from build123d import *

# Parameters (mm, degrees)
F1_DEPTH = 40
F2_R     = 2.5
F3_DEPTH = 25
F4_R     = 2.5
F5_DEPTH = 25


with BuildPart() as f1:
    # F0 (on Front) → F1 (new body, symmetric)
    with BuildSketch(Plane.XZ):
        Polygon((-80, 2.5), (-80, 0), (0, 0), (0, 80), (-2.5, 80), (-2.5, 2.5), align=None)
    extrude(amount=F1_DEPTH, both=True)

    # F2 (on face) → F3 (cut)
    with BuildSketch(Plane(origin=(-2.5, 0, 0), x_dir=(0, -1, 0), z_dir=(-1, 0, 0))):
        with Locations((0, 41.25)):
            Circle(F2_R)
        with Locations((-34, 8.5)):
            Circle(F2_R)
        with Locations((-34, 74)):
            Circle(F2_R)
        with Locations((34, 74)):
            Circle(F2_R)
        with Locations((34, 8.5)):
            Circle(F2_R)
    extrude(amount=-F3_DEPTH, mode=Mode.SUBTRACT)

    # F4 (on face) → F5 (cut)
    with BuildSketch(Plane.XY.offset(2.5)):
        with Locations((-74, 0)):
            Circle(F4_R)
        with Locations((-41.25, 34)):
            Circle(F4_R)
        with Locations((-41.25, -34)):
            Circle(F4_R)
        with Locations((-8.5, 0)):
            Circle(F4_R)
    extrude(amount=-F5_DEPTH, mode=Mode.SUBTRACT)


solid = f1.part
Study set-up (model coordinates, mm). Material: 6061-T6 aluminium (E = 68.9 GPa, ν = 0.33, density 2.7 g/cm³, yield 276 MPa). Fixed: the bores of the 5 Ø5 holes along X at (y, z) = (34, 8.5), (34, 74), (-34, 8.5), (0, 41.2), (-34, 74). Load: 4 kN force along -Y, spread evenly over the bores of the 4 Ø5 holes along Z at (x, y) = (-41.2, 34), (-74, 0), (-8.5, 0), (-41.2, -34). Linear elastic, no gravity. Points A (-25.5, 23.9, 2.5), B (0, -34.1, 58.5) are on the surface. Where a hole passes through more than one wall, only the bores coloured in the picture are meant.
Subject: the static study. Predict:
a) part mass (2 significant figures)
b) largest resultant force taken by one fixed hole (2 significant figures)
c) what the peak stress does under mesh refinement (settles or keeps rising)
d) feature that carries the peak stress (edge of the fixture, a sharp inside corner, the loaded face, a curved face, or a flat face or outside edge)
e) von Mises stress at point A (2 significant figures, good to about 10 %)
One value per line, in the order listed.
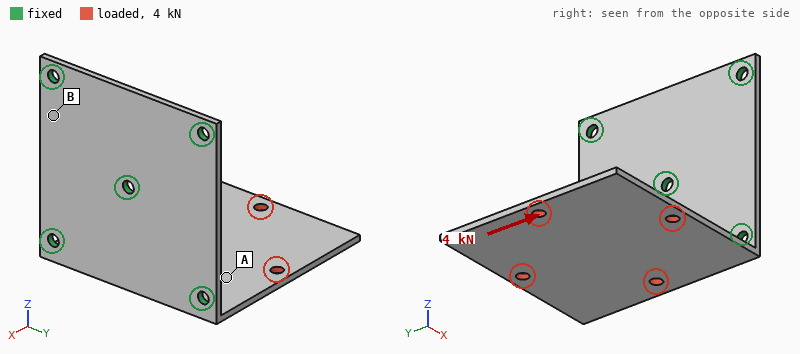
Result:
84 g
3.0 kN
keeps rising
edge of the fixture
58 MPa
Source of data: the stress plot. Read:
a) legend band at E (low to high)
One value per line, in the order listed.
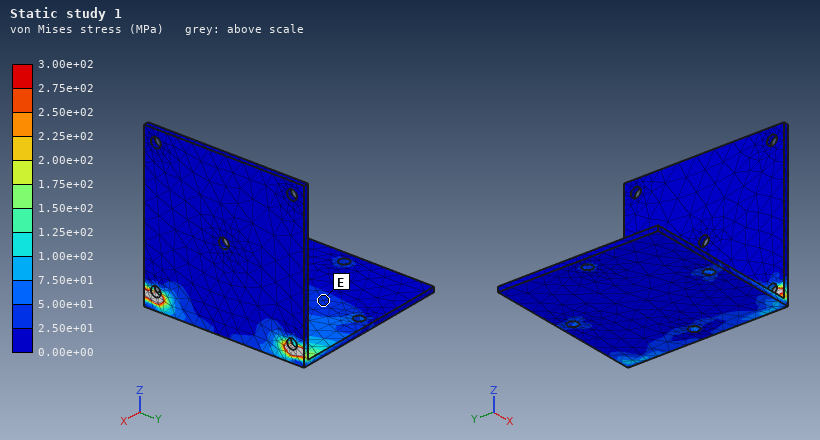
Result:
2.50e+01 to 5.00e+01 MPa
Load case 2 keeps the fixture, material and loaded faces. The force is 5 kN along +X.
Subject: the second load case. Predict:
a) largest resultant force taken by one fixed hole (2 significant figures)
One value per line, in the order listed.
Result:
2.6 kN
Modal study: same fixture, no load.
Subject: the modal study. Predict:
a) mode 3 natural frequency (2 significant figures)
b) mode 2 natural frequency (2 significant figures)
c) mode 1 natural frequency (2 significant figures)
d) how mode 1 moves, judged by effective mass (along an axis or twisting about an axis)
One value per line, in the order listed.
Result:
1800 Hz
760 Hz
290 Hz
along Z
